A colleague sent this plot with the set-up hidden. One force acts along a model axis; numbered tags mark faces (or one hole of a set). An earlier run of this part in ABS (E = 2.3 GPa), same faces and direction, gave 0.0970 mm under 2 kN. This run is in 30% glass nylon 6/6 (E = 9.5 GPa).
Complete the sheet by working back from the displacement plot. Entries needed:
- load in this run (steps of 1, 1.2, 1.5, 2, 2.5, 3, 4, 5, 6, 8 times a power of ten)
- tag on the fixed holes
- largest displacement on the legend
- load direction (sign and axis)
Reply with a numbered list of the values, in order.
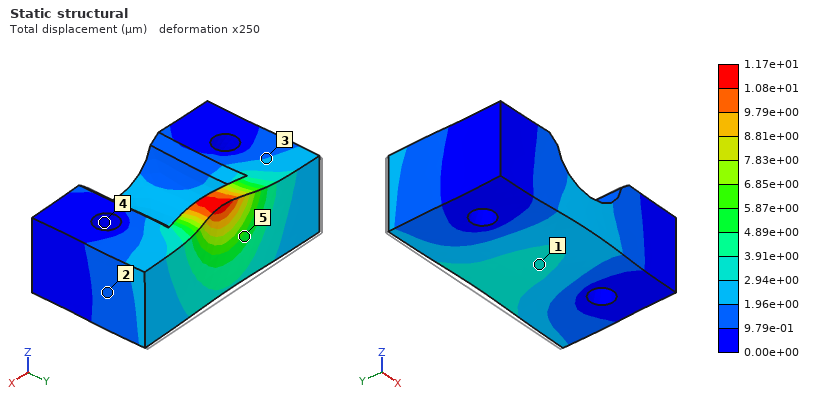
1. 1 kN
2. 4
3. 1.17e+01 µm
4. -Y
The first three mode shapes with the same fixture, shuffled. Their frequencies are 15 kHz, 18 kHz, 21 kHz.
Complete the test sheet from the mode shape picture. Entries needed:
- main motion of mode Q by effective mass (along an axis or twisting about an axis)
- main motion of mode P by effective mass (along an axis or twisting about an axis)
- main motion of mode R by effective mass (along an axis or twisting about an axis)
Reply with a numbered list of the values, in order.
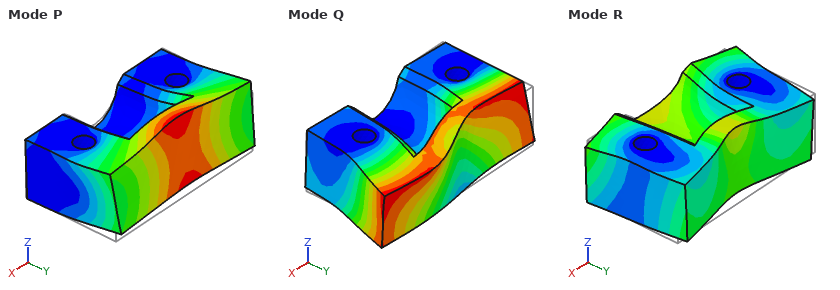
1. along X
2. along Z
3. along Y
